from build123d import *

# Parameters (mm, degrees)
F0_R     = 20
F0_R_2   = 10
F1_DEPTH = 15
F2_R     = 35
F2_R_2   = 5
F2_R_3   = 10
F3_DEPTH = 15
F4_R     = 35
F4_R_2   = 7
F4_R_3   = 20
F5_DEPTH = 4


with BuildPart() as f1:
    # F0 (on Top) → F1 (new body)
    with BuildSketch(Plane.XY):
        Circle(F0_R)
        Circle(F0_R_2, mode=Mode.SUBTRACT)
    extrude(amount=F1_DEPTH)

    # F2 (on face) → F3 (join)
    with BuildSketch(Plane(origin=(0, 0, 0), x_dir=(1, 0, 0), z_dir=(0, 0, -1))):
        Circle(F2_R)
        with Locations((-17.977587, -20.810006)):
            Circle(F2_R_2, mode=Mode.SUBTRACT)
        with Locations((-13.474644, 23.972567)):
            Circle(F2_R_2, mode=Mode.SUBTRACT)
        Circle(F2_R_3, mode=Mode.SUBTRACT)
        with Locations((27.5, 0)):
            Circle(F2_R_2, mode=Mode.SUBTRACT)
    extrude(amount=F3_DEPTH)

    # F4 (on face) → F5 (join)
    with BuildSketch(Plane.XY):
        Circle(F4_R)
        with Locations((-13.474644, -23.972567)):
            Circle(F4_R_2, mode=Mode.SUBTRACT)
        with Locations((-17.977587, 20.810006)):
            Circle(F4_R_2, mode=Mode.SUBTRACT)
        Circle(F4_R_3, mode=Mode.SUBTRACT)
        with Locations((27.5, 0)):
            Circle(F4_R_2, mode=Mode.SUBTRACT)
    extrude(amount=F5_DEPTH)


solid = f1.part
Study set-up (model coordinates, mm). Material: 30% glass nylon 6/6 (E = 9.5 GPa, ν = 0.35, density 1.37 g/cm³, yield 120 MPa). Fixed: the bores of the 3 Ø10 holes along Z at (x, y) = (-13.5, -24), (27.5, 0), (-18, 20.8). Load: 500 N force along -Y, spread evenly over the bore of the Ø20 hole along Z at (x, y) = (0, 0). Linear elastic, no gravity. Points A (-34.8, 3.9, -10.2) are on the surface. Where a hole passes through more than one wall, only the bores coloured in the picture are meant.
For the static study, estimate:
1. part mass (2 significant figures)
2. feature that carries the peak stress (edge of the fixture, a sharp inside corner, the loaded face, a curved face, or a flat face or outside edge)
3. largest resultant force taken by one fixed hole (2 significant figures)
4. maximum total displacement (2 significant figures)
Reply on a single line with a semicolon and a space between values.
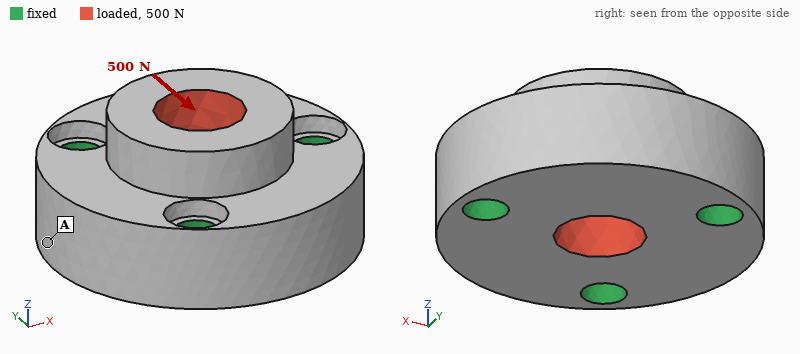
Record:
99 g; edge of the fixture; 180 N; 2.8 µm
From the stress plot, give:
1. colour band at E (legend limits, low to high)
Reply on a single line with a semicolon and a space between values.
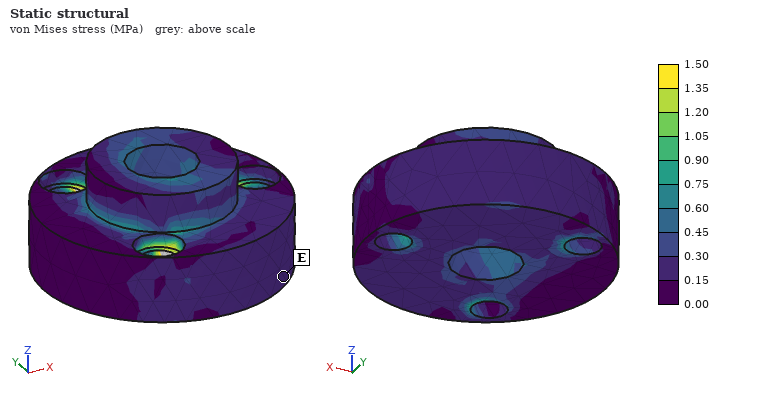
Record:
0.15 to 0.30 MPa
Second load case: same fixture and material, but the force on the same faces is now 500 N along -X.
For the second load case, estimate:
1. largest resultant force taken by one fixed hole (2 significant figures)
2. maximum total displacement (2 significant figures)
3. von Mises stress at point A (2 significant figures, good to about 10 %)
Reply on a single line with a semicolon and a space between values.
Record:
190 N; 2.7 µm; 0.28 MPa
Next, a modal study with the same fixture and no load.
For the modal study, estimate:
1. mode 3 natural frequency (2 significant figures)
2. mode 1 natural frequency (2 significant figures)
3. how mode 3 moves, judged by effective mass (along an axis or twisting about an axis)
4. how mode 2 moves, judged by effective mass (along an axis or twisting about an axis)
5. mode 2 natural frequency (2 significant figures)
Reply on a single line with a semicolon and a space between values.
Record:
11 kHz; 8500 Hz; along Z; along Z; 9900 Hz
